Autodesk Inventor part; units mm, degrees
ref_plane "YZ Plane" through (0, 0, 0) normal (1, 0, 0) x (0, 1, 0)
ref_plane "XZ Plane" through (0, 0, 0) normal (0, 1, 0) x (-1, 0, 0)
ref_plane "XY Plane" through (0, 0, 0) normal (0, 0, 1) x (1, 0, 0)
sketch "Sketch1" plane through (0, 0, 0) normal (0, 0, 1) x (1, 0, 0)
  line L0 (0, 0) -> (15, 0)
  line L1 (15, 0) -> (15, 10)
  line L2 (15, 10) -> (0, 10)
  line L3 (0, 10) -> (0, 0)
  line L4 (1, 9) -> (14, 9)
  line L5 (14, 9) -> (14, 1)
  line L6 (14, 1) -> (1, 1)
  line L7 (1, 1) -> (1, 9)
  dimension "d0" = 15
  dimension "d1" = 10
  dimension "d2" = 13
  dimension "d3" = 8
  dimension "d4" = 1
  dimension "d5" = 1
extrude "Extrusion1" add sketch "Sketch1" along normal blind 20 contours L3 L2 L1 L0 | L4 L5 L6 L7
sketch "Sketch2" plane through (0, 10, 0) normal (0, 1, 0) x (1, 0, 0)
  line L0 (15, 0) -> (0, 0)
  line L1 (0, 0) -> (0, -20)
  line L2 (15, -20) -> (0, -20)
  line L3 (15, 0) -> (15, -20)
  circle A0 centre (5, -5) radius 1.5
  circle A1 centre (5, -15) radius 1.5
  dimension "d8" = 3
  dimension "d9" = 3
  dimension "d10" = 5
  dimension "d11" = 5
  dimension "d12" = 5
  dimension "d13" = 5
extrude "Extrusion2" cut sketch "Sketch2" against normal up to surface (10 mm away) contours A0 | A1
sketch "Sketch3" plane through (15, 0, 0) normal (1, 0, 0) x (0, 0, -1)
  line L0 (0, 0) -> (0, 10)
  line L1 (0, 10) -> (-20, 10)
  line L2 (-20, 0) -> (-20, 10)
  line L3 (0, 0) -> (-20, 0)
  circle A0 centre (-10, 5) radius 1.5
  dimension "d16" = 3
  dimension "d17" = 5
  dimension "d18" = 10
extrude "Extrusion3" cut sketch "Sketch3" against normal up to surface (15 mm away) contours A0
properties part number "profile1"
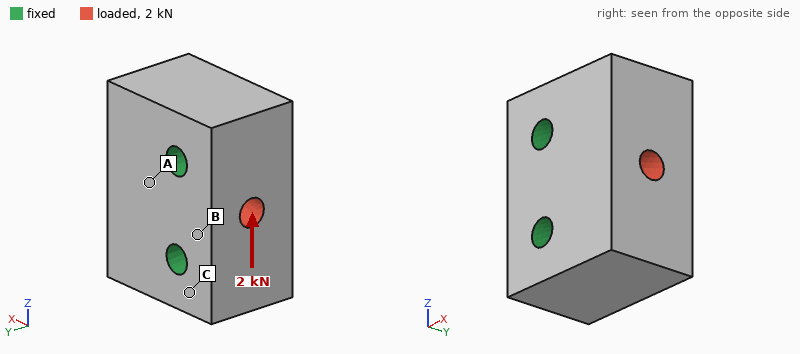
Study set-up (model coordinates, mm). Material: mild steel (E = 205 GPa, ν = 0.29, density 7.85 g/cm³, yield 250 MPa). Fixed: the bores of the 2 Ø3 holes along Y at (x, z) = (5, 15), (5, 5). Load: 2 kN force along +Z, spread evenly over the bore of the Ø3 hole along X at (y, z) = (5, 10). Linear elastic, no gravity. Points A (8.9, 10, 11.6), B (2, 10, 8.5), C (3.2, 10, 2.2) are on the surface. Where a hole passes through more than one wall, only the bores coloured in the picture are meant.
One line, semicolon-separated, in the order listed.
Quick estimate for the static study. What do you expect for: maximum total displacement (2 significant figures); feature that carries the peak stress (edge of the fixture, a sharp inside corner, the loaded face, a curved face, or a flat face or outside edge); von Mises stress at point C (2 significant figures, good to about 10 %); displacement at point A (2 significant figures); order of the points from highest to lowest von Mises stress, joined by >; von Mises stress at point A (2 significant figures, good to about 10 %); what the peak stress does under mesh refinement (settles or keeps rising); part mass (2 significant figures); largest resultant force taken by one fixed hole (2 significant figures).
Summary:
0.87 µm; edge of the fixture; 6.1 MPa; 0.29 µm; A > C > B; 11 MPa; keeps rising; 22 g; 1.1 kN
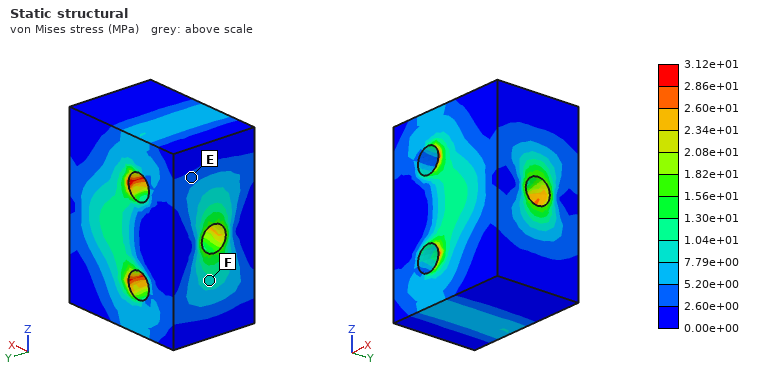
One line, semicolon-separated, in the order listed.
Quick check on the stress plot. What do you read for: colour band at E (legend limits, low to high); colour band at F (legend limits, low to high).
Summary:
2.60e+00 to 5.20e+00 MPa; 7.79e+00 to 1.04e+01 MPa
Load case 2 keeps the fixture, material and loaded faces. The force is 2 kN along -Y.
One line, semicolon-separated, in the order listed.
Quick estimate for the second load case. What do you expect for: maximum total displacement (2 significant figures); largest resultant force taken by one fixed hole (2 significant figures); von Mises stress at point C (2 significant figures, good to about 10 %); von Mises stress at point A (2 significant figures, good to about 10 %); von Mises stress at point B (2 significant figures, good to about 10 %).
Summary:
1.5 µm; 1.0 kN; 7.8 MPa; 11 MPa; 9.1 MPa
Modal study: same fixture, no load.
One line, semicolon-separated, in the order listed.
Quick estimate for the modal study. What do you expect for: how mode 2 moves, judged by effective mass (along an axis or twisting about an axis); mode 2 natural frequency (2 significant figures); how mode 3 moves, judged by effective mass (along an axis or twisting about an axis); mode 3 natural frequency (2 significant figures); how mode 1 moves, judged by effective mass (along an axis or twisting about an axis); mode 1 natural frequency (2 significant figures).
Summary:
along Z; 59 kHz; twisting about X; 67 kHz; along Y; 53 kHz
